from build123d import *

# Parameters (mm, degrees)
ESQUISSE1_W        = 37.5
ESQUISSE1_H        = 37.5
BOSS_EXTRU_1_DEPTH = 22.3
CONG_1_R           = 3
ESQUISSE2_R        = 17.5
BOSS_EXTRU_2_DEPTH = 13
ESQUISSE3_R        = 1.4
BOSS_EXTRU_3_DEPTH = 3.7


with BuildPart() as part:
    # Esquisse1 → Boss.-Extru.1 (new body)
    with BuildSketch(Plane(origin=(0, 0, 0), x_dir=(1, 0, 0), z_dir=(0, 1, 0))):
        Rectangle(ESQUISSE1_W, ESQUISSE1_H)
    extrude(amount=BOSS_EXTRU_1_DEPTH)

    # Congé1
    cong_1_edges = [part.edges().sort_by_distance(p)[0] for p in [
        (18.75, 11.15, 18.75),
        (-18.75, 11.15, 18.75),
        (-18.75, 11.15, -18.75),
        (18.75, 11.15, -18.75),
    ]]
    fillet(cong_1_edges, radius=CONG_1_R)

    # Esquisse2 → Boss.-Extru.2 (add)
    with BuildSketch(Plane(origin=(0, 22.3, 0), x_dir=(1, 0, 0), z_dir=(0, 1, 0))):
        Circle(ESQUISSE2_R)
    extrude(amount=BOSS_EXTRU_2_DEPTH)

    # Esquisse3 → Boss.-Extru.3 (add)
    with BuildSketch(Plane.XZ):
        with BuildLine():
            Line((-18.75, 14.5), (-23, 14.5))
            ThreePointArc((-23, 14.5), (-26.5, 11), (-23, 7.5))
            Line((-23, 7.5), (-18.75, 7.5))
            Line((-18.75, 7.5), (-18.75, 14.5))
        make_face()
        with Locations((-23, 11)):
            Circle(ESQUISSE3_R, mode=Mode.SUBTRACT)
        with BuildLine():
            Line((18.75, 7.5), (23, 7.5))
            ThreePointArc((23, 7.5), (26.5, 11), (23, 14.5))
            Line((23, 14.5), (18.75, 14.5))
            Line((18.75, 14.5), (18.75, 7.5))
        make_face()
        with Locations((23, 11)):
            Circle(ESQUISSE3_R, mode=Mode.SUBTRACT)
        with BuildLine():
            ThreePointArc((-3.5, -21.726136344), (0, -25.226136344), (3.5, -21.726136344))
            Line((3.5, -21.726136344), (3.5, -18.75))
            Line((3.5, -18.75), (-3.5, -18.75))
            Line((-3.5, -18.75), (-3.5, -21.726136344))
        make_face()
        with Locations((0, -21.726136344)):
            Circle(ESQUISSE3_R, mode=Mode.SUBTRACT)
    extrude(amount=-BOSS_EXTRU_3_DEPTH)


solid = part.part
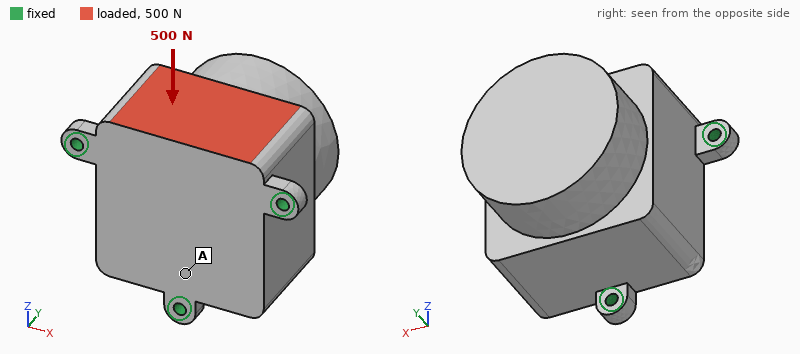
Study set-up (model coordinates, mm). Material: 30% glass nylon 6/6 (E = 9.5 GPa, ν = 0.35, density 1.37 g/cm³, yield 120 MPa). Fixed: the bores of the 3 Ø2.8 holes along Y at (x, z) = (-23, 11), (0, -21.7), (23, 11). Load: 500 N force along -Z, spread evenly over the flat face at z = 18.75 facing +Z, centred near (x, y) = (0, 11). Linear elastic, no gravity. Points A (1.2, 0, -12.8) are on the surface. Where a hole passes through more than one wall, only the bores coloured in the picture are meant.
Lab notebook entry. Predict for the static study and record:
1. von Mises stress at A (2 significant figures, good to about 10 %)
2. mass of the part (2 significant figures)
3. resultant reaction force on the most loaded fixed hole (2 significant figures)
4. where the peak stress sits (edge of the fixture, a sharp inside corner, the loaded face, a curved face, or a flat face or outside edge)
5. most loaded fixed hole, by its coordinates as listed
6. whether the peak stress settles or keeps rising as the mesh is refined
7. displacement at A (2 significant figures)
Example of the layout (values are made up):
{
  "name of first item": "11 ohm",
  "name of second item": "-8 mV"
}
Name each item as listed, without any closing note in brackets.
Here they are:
{
  "von Mises stress at A": "2.8 MPa",
  "mass of the part": "60 g",
  "resultant reaction force on the most loaded fixed hole": "340 N",
  "where the peak stress sits": "edge of the fixture",
  "most loaded fixed hole, by its coordinates as listed": "(0, -21.7)",
  "whether the peak stress settles or keeps rising as the mesh is refined": "keeps rising",
  "displacement at A": "6.6 µm"
}
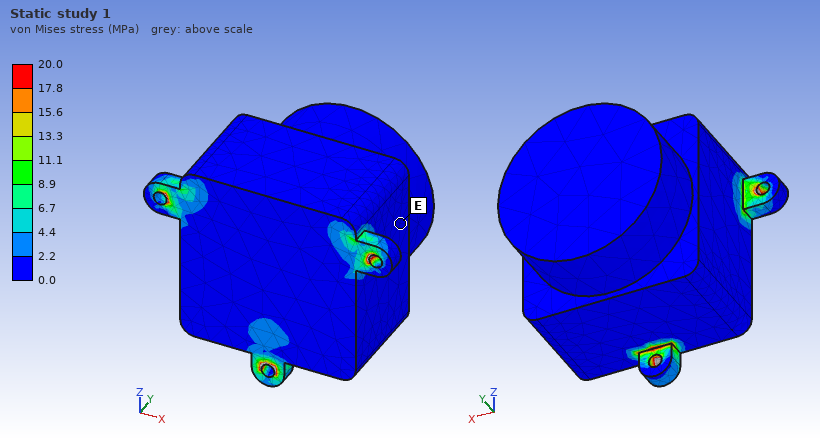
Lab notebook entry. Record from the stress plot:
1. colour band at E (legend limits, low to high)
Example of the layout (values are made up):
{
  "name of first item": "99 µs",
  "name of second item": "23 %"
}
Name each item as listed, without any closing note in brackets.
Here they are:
{
  "colour band at E": "0.0 to 2.2 MPa"
}
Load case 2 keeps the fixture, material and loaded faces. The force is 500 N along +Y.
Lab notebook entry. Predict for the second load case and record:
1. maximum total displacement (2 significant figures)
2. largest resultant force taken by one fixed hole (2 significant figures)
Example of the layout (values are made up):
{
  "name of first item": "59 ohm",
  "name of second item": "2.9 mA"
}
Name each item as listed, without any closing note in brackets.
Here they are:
{
  "maximum total displacement": "67 µm",
  "largest resultant force taken by one fixed hole": "340 N"
}
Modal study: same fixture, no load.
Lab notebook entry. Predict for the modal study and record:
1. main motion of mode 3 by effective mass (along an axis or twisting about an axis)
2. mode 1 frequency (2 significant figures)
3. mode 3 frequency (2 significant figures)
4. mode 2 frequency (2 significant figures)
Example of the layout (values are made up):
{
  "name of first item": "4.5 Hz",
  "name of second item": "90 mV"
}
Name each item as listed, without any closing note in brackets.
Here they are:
{
  "main motion of mode 3 by effective mass": "along Y",
  "mode 1 frequency": "2600 Hz",
  "mode 3 frequency": "3700 Hz",
  "mode 2 frequency": "2600 Hz"
}
